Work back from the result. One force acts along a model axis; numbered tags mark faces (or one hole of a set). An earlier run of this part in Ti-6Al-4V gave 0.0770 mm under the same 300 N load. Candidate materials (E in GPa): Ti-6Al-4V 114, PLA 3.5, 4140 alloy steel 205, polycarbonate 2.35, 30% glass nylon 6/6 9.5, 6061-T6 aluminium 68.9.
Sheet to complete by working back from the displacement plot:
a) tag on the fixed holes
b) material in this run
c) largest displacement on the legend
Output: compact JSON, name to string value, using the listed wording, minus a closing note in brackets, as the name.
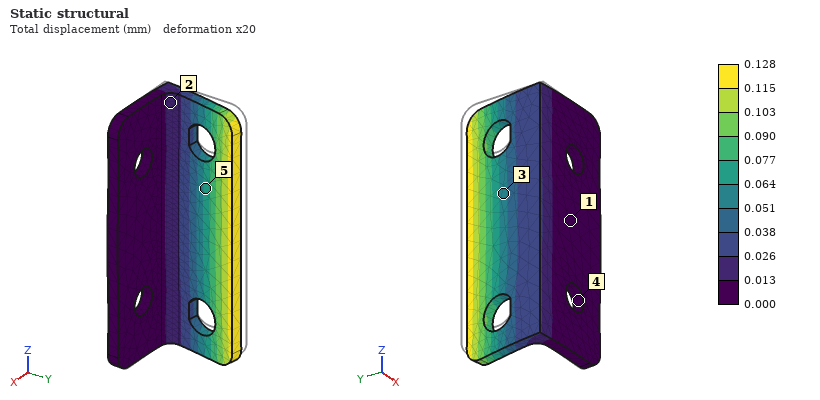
{"tag on the fixed holes": "4", "material in this run": "6061-T6 aluminium", "largest displacement on the legend": "0.128 mm"}
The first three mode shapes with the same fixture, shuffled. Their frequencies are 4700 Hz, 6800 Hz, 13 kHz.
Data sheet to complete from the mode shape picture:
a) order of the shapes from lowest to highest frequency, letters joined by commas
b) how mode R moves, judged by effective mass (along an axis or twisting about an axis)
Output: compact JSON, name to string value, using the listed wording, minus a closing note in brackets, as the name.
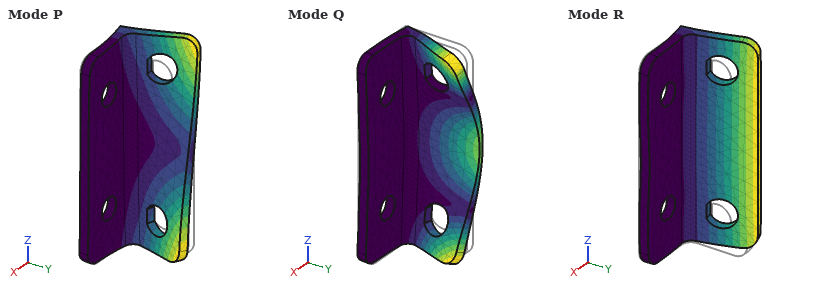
{"order of the shapes from lowest to highest frequency, letters joined by commas": "R, P, Q", "how mode R moves, judged by effective mass": "along X"}
